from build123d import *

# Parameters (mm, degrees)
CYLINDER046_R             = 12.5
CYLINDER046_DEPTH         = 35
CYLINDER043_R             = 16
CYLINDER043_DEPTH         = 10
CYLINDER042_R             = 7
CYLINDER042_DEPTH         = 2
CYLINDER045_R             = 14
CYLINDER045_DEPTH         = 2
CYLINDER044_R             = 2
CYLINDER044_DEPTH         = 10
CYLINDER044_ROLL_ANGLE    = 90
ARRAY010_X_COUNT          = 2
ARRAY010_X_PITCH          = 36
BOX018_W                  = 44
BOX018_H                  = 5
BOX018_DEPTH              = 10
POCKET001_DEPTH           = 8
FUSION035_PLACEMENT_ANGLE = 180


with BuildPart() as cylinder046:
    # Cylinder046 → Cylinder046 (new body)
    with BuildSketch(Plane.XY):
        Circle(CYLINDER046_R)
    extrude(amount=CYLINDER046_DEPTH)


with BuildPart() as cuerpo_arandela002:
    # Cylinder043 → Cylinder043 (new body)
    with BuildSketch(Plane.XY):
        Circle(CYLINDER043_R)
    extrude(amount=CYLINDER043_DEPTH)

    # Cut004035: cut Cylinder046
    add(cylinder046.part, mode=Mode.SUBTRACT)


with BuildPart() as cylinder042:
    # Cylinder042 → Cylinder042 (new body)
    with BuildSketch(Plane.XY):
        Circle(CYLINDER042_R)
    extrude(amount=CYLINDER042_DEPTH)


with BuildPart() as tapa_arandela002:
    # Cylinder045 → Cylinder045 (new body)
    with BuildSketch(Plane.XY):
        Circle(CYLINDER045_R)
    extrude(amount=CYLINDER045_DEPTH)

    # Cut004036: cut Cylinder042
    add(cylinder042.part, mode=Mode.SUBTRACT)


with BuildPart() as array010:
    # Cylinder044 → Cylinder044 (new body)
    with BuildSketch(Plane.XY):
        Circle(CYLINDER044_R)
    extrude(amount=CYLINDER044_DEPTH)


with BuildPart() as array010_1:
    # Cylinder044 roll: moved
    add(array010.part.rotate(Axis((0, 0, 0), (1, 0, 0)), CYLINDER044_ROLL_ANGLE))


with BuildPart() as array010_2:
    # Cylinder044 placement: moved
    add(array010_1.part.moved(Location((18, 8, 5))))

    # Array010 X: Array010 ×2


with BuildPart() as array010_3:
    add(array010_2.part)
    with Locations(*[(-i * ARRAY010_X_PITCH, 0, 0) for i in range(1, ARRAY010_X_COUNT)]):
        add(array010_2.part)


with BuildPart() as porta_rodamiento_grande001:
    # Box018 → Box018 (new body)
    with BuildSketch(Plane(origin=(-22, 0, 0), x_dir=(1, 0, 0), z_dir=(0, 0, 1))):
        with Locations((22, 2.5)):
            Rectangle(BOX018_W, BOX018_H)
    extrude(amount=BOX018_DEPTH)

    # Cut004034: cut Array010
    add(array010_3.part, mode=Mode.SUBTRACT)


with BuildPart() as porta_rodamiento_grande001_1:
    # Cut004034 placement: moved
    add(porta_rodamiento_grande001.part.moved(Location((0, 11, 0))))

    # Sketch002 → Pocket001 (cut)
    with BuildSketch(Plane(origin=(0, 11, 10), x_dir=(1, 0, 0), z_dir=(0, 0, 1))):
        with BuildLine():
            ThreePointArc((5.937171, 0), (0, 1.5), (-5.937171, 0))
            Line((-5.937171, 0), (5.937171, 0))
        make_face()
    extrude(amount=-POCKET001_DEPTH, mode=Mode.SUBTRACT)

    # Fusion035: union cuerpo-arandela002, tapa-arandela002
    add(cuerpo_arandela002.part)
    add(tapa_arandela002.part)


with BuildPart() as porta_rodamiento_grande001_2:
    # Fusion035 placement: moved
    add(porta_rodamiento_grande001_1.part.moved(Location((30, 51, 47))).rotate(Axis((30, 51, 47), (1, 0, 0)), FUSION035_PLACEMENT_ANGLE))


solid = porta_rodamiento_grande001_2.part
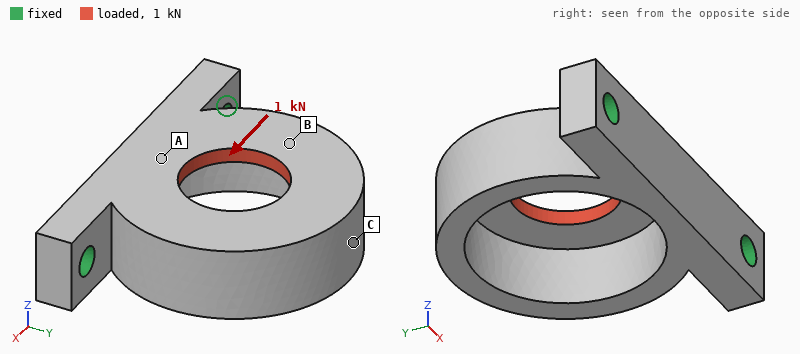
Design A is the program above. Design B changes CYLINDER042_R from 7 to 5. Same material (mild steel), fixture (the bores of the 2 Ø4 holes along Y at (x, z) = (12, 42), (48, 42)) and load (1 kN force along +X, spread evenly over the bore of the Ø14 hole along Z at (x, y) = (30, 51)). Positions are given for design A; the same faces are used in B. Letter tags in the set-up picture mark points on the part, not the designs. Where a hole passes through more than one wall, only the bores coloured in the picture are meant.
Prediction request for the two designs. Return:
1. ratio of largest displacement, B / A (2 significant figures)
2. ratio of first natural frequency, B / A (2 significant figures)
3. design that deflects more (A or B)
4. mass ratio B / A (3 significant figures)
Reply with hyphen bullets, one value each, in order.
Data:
- 0.81
- 0.99
- A
- 1.03
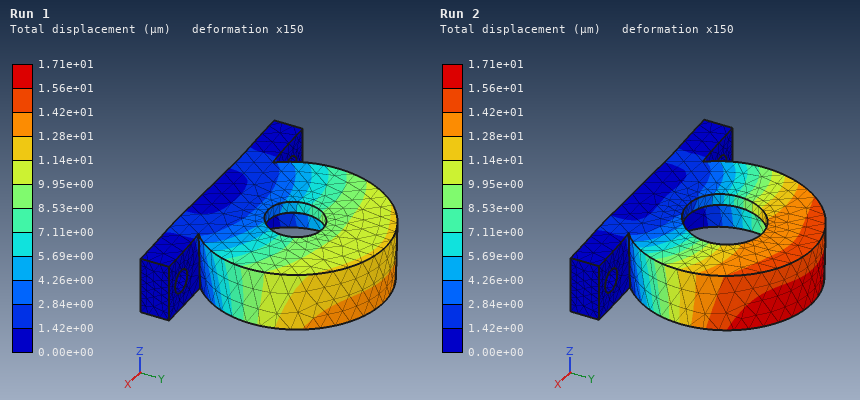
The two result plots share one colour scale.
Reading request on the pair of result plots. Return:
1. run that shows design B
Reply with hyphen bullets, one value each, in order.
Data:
- Run 1
